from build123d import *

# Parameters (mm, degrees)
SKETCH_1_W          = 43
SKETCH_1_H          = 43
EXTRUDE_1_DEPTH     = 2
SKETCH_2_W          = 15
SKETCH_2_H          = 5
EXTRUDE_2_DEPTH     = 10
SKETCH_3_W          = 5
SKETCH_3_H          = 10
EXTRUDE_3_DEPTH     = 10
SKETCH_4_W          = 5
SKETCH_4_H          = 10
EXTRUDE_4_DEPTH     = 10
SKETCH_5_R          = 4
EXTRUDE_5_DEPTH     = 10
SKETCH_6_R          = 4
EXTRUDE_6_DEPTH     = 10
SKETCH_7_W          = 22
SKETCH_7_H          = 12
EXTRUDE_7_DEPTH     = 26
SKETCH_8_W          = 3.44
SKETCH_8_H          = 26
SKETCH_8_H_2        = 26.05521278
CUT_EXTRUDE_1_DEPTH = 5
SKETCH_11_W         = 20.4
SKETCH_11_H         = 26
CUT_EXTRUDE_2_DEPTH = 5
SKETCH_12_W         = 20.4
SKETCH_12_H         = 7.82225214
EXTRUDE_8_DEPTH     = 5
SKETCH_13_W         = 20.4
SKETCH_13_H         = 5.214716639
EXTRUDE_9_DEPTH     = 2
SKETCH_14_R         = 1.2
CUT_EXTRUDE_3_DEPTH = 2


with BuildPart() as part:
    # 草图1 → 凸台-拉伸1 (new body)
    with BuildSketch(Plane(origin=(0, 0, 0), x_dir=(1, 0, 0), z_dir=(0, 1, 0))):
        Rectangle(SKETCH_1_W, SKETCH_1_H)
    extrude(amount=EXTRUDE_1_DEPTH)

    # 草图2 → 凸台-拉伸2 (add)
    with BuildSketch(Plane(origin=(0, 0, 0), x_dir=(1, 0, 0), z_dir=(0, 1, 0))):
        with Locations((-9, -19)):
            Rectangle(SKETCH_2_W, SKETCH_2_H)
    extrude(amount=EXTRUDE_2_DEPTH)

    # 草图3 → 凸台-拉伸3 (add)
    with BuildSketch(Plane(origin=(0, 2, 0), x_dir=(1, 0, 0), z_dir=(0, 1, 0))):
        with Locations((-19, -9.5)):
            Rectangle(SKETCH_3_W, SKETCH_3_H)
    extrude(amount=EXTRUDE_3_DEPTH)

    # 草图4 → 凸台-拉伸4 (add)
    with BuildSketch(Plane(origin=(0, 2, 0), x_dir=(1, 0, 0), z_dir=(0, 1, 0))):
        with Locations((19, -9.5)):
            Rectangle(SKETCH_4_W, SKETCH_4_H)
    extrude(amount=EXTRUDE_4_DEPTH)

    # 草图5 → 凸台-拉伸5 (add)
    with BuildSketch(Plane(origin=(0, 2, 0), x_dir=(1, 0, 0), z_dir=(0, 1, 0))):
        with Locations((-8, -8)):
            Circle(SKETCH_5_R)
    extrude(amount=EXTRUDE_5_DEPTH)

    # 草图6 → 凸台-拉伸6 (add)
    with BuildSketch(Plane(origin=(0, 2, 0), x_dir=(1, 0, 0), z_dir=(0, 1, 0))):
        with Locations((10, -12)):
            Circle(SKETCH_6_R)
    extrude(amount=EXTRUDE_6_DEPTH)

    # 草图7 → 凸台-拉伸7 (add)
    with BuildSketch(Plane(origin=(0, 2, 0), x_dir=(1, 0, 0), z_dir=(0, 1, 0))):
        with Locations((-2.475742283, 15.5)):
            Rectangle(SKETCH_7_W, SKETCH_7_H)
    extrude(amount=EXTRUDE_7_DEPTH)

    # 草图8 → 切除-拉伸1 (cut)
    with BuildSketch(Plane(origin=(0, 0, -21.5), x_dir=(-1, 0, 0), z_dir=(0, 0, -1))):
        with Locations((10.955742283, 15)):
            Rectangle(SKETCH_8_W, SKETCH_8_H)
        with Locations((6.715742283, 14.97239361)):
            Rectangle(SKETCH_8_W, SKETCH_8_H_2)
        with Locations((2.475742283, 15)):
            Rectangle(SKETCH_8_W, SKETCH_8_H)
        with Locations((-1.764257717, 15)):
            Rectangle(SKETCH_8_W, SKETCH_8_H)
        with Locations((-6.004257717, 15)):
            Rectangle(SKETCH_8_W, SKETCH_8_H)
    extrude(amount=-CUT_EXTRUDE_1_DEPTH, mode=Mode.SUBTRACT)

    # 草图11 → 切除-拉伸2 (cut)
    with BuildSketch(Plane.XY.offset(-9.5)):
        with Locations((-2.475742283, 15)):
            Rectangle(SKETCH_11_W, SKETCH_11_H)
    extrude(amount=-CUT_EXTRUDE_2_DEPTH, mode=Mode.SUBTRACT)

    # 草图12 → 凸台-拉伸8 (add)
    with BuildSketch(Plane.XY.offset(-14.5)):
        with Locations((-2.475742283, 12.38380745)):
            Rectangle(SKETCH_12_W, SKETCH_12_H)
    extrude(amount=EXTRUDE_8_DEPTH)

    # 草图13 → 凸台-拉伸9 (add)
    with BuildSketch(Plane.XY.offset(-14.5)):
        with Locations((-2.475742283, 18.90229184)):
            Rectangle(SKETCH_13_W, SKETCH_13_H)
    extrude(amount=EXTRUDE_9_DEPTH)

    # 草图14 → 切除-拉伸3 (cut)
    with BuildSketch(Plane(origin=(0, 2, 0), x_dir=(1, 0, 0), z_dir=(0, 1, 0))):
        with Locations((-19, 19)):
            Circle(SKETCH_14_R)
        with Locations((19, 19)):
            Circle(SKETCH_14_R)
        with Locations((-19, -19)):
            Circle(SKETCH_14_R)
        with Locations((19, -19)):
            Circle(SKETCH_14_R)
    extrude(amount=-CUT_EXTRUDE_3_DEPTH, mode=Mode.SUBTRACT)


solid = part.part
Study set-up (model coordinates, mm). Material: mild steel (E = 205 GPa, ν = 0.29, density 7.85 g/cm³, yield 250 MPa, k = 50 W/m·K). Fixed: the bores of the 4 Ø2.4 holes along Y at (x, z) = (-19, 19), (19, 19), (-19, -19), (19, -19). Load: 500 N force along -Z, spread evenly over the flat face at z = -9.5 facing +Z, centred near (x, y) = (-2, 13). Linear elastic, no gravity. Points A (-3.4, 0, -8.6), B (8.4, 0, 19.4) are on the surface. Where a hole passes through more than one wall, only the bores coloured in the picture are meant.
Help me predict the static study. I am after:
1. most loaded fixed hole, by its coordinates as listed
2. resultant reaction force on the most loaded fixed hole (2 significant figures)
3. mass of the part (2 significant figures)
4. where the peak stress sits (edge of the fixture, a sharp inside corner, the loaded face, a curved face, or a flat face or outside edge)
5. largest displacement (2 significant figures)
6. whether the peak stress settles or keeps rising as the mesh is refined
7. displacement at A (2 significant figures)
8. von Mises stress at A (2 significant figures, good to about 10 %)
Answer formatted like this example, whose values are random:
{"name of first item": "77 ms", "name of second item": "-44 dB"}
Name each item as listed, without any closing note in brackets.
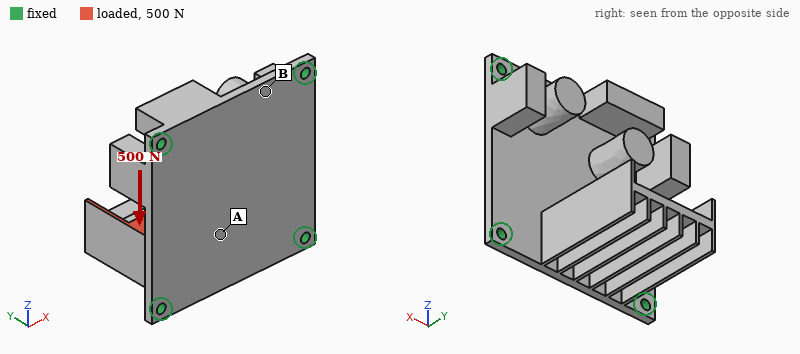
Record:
{"most loaded fixed hole, by its coordinates as listed": "(-19, -19)", "resultant reaction force on the most loaded fixed hole": "220 N", "mass of the part": "73 g", "where the peak stress sits": "edge of the fixture", "largest displacement": "0.13 mm", "whether the peak stress settles or keeps rising as the mesh is refined": "keeps rising", "displacement at A": "0.025 mm", "von Mises stress at A": "71 MPa"}
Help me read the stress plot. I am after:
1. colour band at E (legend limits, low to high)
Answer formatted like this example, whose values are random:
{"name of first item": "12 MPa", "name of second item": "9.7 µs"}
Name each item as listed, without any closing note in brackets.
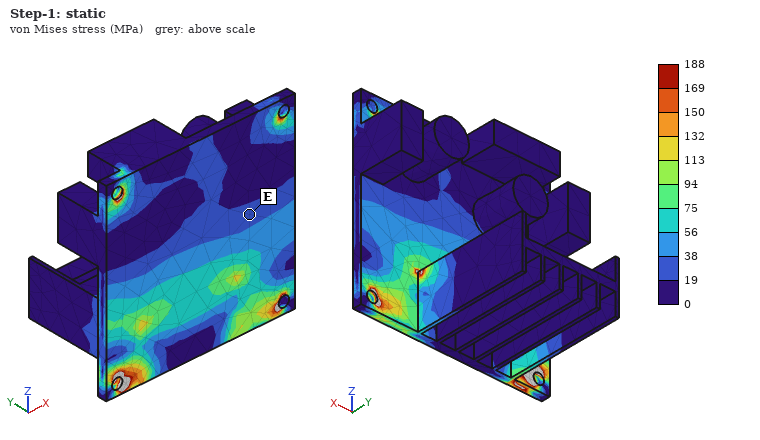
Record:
{"colour band at E": "19 to 38 MPa"}
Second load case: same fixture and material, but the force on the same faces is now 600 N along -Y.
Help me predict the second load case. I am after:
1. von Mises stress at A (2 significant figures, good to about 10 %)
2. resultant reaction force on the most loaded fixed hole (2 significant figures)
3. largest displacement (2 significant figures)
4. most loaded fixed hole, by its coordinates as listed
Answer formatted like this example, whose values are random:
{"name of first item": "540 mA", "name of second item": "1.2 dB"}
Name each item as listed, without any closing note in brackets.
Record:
{"von Mises stress at A": "61 MPa", "resultant reaction force on the most loaded fixed hole": "280 N", "largest displacement": "91 µm", "most loaded fixed hole, by its coordinates as listed": "(-19, -19)"}
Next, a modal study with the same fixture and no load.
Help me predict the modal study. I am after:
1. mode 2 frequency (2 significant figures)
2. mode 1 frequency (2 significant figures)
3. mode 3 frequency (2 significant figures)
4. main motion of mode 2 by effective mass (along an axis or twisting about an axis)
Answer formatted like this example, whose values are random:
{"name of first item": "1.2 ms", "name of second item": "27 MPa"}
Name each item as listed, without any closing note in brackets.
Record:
{"mode 2 frequency": "4000 Hz", "mode 1 frequency": "2300 Hz", "mode 3 frequency": "5200 Hz", "main motion of mode 2 by effective mass": "along Y"}
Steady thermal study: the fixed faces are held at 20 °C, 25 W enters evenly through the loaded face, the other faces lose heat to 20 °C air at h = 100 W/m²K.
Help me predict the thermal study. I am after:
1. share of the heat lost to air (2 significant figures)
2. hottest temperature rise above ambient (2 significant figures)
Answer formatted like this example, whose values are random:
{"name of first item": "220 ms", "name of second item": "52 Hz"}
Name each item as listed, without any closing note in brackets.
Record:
{"share of the heat lost to air": "76 %", "hottest temperature rise above ambient": "64 K"}
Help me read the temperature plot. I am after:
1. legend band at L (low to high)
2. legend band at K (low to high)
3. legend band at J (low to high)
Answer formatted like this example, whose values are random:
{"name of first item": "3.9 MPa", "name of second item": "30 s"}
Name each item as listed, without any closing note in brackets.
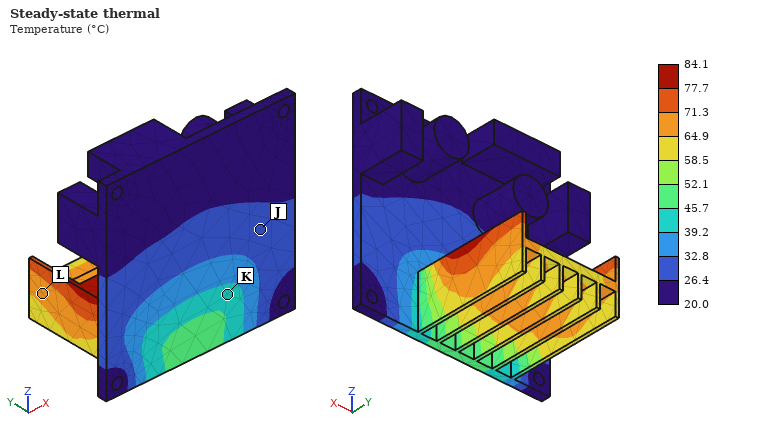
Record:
{"legend band at L": "64.9 to 71.3 °C", "legend band at K": "39.2 to 45.7 °C", "legend band at J": "26.4 to 32.8 °C"}
